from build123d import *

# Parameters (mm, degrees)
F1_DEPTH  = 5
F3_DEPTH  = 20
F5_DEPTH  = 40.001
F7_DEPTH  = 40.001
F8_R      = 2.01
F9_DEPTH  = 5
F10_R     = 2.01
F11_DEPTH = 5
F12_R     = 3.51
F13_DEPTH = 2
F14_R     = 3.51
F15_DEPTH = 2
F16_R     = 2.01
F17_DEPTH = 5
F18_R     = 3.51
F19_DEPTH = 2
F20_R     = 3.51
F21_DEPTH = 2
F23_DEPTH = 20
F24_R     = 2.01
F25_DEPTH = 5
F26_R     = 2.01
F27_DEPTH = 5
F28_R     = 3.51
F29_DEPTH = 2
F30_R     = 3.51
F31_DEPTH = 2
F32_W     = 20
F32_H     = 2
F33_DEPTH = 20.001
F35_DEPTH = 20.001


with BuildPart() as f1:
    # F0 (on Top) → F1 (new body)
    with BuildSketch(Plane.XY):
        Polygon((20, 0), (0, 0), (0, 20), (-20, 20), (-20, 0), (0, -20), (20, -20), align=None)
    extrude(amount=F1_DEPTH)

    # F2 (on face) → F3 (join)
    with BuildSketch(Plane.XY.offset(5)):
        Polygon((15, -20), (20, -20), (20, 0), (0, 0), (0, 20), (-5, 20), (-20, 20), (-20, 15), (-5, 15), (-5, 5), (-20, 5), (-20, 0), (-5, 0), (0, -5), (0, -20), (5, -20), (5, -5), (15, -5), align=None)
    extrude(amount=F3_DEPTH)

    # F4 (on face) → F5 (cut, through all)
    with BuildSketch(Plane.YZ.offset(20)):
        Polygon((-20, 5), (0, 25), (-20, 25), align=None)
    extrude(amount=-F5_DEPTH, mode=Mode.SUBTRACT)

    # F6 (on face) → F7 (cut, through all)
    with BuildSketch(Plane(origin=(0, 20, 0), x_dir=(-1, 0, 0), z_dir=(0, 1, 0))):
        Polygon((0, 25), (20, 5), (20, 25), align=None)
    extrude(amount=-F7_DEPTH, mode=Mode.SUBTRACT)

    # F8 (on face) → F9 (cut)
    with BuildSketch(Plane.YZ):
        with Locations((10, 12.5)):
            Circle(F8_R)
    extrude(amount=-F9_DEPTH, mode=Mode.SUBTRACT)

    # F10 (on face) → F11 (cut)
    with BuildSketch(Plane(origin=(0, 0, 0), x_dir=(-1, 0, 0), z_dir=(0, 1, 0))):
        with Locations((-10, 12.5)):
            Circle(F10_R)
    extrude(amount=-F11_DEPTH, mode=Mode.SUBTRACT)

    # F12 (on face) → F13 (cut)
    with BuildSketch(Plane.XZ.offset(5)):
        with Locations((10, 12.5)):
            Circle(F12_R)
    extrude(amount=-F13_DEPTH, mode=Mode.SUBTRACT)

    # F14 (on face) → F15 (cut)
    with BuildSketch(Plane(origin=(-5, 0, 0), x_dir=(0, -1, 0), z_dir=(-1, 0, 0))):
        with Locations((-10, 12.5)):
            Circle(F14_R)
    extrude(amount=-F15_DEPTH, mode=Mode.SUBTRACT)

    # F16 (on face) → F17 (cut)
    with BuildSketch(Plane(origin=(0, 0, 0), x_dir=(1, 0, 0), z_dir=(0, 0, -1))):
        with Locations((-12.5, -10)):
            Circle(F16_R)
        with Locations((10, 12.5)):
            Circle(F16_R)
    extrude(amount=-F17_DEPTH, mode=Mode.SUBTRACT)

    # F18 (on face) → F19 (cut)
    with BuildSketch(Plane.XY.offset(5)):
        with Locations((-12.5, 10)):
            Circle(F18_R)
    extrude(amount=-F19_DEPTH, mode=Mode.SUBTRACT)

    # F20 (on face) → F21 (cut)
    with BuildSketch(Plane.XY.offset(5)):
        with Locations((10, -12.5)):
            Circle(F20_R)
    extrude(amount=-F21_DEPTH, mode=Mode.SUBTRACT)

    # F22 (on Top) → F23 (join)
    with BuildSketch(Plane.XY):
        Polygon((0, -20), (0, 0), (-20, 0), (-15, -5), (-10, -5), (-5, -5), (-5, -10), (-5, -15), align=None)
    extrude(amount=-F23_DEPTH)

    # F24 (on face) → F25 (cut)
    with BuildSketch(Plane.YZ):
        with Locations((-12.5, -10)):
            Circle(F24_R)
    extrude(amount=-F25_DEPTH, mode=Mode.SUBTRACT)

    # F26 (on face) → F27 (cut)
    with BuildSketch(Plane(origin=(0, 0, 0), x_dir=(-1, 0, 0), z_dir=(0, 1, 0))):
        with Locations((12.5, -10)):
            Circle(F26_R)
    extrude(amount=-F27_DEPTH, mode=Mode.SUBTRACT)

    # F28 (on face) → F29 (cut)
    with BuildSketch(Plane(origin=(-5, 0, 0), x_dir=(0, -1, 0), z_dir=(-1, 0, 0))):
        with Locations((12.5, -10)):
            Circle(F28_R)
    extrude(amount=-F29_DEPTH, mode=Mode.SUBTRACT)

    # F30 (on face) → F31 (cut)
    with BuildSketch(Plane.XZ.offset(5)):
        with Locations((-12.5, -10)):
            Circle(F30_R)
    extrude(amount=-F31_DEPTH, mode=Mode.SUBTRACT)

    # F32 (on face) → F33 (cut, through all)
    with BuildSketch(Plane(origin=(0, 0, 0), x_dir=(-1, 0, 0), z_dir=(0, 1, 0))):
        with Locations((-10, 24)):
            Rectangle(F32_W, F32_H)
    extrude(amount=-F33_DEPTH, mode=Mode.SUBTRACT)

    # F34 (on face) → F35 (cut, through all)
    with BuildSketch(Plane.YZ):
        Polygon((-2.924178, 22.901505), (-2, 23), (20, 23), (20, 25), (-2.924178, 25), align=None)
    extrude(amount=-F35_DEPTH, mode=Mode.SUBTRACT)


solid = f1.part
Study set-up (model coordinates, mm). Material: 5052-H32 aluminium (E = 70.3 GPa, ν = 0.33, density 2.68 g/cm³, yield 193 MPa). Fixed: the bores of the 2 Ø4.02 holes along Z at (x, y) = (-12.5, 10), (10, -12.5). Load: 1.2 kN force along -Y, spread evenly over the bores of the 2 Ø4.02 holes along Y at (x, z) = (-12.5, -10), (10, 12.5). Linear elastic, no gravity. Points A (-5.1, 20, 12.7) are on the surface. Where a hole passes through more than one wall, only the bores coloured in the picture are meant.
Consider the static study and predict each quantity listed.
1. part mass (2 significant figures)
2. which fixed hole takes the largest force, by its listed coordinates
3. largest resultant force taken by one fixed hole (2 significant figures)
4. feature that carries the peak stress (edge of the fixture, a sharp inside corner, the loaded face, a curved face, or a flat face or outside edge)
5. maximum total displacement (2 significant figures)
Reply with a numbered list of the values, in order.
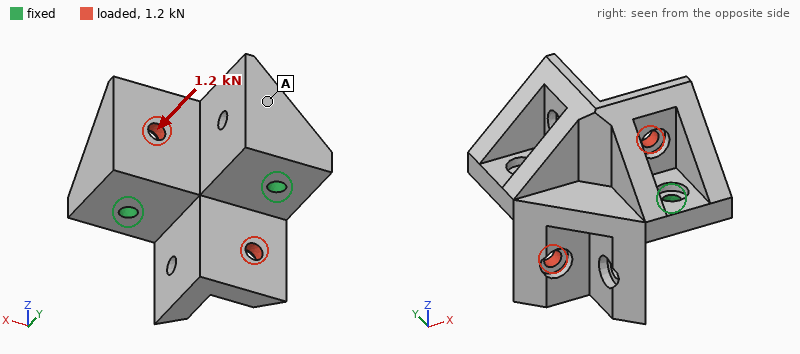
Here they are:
1. 35 g
2. (-12.5, 10)
3. 690 N
4. a curved face
5. 49 µm
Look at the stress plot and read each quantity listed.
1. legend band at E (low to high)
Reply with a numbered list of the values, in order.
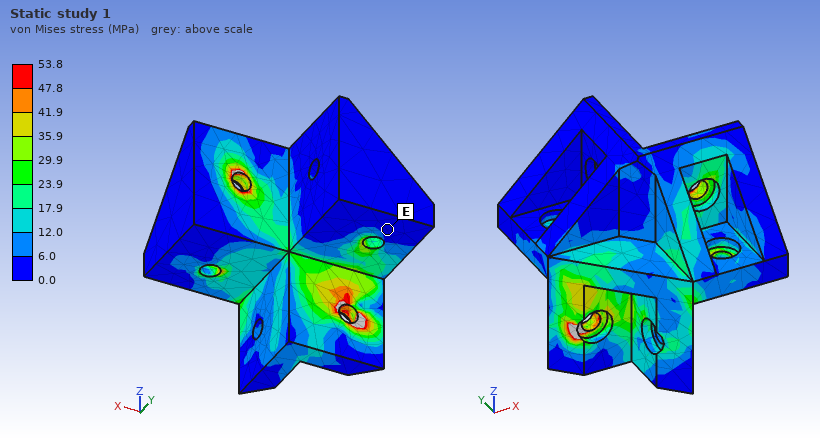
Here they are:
1. 0.0 to 6.0 MPa
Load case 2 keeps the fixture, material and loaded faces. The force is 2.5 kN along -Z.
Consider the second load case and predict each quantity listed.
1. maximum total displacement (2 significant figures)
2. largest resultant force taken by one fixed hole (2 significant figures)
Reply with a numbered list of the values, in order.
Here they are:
1. 38 µm
2. 1.4 kN
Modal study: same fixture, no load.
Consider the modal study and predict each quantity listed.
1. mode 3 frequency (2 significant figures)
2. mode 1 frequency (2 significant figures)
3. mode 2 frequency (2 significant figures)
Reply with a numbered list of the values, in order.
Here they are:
1. 12 kHz
2. 4500 Hz
3. 11 kHz
